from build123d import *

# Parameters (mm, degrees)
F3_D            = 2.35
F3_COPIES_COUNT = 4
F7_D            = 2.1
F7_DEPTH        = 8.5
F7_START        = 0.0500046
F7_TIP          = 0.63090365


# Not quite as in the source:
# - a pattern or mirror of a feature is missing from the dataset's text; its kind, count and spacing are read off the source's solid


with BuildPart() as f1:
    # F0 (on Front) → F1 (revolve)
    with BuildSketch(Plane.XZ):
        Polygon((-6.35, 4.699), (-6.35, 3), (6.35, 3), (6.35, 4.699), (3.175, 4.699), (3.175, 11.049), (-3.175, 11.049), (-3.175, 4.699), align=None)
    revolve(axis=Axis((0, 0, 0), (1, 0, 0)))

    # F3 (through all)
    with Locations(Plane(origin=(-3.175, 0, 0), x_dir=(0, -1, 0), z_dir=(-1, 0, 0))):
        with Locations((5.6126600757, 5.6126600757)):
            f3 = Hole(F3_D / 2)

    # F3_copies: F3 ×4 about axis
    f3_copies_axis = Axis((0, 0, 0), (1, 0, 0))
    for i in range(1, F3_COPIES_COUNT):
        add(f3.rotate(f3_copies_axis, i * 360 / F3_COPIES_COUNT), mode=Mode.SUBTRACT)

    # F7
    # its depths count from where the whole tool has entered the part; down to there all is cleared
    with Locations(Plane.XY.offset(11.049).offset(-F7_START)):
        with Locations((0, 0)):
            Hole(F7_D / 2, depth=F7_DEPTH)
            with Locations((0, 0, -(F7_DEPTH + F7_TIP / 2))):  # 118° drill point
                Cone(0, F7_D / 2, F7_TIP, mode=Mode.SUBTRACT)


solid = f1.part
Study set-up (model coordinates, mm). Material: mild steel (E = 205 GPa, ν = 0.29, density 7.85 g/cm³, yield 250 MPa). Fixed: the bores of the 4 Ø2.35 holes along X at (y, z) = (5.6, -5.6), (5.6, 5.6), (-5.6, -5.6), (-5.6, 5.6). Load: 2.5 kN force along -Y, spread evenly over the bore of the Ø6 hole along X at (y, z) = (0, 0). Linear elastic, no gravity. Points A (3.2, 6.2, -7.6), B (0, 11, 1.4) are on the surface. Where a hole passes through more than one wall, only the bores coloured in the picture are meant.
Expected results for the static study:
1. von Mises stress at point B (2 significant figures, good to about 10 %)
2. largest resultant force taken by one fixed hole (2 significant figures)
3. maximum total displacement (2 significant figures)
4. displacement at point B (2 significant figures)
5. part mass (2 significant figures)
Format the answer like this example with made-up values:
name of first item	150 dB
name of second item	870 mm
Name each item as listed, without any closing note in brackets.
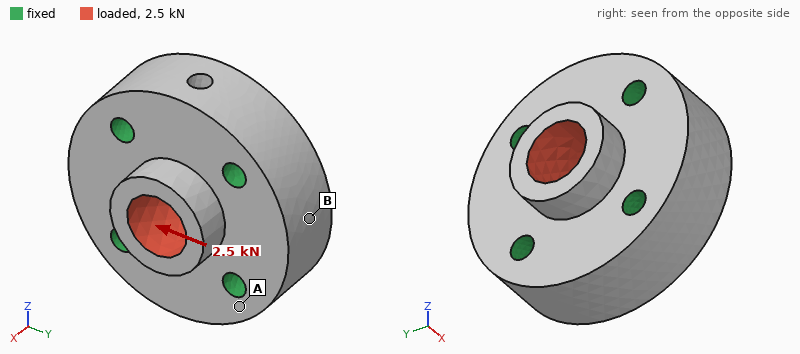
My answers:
von Mises stress at point B	9.1 MPa
largest resultant force taken by one fixed hole	660 N
maximum total displacement	1.7 µm
displacement at point B	0.30 µm
part mass	19 g
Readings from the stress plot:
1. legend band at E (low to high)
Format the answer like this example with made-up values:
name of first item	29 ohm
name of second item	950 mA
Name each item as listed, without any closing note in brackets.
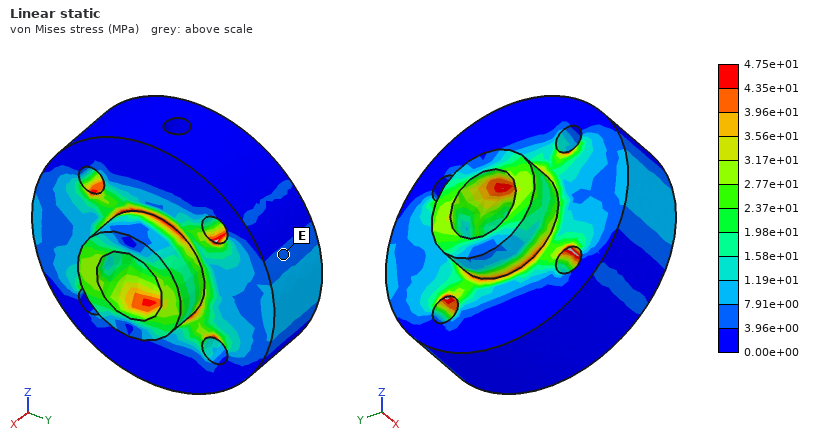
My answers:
legend band at E	3.96e+00 to 7.91e+00 MPa
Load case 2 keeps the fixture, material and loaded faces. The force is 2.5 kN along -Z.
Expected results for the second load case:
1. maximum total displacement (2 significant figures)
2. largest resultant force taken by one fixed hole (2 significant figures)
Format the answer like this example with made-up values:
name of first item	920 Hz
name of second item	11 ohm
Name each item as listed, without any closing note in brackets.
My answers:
maximum total displacement	1.7 µm
largest resultant force taken by one fixed hole	650 N
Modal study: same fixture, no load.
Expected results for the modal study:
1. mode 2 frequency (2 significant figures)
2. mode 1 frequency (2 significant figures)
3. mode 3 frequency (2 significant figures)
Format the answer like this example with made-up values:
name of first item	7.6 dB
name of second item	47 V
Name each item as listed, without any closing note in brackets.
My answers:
mode 2 frequency	96 kHz
mode 1 frequency	95 kHz
mode 3 frequency	97 kHz
